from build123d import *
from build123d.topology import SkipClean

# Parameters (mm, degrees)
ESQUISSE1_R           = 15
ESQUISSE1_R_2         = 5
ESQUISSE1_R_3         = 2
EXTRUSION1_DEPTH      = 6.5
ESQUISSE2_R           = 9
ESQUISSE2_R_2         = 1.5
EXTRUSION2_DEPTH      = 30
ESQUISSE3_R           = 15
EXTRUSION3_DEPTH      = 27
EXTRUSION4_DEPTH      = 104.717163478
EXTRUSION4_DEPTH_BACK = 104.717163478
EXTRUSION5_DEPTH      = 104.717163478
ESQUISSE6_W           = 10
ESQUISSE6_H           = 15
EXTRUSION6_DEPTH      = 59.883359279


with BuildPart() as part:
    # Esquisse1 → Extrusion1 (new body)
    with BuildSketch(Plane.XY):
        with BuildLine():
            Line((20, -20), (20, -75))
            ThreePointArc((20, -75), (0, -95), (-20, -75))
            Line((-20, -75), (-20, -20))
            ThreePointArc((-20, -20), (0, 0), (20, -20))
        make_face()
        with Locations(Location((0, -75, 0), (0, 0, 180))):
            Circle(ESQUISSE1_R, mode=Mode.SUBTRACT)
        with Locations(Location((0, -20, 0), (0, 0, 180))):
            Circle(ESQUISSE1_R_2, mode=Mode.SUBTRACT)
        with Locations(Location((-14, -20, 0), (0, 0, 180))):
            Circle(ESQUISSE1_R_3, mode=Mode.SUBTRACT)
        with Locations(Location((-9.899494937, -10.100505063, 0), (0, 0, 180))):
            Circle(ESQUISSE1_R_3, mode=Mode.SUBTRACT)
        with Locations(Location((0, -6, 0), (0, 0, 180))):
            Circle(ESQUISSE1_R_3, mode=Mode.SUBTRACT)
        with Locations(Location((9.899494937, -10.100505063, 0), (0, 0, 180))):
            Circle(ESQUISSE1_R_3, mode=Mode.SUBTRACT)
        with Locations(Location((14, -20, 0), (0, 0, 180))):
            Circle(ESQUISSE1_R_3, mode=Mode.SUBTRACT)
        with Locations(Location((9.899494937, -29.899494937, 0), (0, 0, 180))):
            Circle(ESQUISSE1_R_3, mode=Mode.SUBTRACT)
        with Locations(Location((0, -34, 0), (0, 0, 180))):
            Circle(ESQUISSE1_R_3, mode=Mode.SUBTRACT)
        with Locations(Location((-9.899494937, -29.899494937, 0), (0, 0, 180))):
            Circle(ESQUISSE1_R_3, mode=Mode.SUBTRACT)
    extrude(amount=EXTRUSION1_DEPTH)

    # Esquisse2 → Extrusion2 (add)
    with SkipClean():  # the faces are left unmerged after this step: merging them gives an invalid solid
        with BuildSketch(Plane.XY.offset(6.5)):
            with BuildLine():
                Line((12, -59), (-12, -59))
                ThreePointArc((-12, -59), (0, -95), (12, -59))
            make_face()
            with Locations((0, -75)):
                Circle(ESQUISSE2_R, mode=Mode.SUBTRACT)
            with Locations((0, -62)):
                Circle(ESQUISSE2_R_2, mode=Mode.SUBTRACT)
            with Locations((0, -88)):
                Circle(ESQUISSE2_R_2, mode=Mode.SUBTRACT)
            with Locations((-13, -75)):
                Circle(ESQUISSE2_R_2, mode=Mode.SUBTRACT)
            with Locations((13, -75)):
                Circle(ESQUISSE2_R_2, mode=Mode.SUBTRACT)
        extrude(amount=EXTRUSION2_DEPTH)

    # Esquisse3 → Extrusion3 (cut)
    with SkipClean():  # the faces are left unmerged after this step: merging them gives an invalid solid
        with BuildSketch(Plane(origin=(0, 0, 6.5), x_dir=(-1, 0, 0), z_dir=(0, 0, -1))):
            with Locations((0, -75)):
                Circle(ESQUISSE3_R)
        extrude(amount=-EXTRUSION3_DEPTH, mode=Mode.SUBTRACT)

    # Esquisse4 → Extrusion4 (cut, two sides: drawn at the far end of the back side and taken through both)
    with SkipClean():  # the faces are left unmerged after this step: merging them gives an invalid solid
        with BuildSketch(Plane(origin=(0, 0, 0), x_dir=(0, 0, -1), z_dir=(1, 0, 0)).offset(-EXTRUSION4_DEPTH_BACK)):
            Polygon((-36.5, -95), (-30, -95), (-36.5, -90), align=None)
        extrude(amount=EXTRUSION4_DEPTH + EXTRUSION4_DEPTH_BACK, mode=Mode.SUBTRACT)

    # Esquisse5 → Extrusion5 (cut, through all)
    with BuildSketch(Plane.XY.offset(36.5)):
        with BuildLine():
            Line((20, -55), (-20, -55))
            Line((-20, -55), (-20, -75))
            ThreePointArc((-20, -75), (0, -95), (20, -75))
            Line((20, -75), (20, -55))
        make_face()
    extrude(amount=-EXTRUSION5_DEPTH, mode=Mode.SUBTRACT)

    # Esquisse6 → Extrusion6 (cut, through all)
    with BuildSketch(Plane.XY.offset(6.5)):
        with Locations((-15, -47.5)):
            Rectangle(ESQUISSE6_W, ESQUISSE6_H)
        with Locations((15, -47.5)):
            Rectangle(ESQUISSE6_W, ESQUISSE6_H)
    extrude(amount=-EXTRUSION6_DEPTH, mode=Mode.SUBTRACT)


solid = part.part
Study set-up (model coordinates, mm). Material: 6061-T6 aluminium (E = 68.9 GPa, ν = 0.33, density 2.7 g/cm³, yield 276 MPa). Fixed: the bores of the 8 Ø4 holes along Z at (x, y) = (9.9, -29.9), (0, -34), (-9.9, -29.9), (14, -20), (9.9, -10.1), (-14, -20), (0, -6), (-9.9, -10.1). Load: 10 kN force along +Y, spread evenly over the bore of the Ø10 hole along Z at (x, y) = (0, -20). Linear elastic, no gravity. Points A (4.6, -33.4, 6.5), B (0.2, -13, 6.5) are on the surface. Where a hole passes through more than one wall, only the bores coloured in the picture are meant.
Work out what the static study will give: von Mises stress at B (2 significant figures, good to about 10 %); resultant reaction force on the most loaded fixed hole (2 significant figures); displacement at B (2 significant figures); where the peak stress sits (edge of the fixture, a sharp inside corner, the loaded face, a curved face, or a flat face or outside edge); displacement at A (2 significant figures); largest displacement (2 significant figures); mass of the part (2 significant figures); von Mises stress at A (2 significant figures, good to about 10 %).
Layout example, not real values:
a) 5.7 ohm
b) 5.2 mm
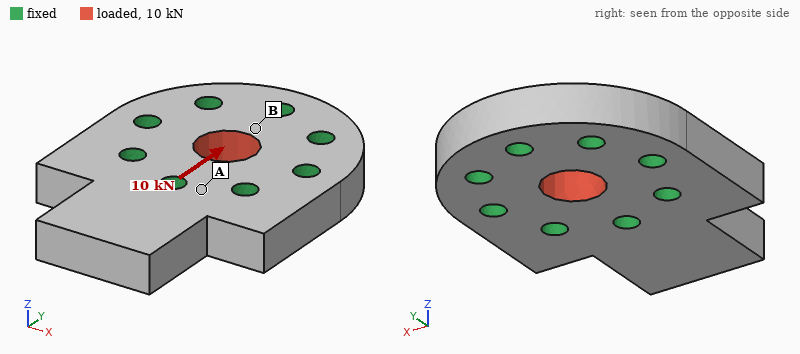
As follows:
a) 47 MPa
b) 2.1 kN
c) 3.8 µm
d) the loaded face
e) 1.0 µm
f) 5.6 µm
g) 27 g
h) 14 MPa
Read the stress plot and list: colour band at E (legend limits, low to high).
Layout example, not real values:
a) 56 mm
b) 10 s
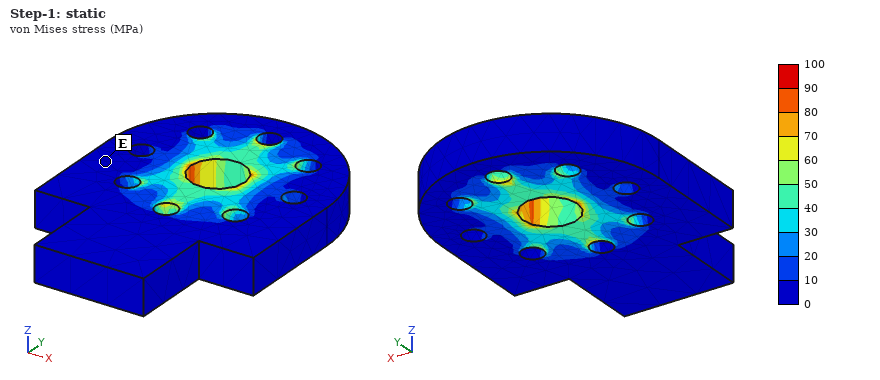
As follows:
a) 0 to 10 MPa
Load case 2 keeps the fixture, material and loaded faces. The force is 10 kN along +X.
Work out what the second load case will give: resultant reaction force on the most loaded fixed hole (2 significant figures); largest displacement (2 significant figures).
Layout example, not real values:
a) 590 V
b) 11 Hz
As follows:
a) 2.1 kN
b) 5.6 µm
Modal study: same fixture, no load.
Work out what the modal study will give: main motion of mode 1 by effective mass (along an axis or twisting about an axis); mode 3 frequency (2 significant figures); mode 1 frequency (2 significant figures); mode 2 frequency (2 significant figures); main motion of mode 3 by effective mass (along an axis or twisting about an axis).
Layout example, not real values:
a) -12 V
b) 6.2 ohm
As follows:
a) along Z
b) 27 kHz
c) 12 kHz
d) 24 kHz
e) along X
